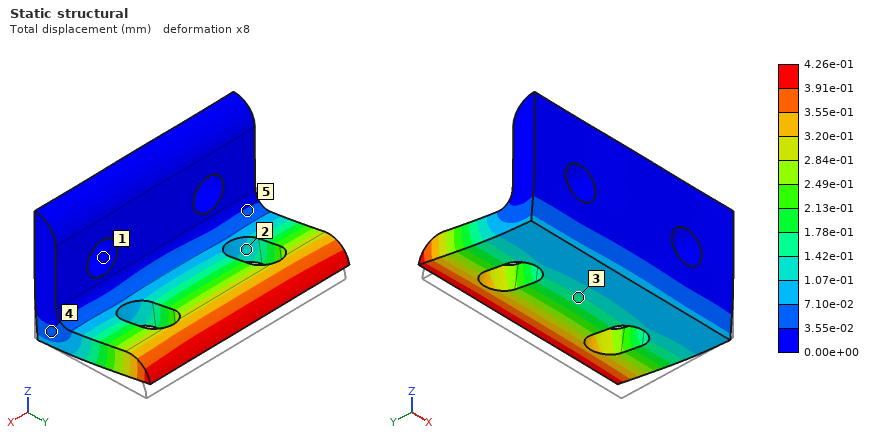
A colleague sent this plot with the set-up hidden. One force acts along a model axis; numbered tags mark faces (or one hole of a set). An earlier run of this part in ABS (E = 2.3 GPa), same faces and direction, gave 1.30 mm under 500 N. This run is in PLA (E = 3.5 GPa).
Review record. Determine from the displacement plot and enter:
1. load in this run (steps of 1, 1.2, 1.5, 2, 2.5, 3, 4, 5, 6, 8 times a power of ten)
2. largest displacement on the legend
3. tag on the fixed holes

250 N
4.26e-01 mm
1
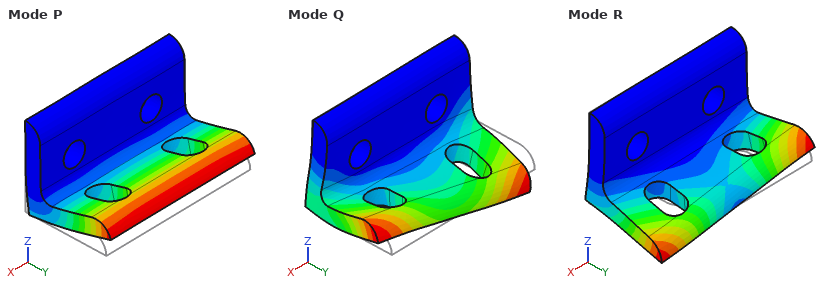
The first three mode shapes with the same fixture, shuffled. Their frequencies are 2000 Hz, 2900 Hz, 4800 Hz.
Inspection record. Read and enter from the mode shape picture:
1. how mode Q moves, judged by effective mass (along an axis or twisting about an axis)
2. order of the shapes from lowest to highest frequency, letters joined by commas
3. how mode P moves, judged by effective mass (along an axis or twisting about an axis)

along X
P, R, Q
along Z
